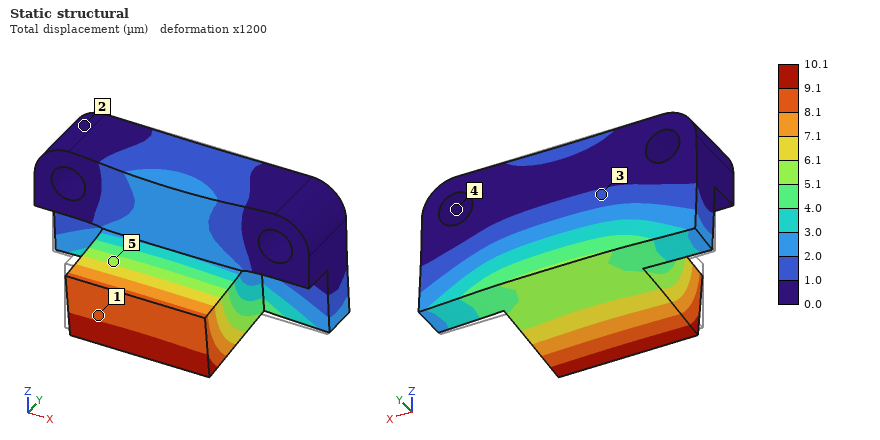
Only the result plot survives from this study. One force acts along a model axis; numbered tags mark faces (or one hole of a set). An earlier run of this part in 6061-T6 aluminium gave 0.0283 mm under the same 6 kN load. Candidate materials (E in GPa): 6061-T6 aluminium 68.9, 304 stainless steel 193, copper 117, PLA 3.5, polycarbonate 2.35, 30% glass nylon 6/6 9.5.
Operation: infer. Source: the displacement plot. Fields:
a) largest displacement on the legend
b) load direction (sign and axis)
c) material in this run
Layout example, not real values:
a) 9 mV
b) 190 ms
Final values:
a) 10.1 µm
b) -Z
c) 304 stainless steel
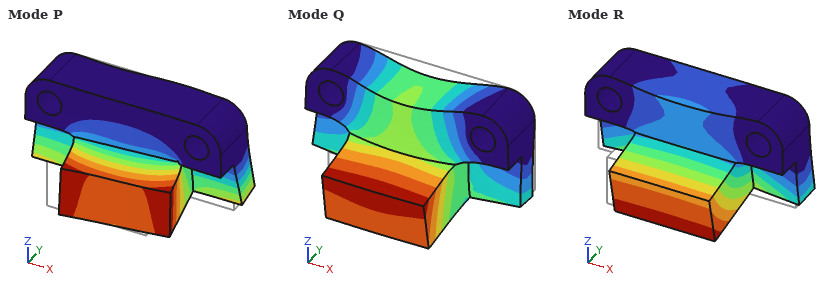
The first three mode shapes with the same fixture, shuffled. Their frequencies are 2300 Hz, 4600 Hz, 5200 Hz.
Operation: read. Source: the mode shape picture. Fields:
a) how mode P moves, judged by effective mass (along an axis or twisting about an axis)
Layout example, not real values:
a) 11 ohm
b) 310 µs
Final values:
a) along X
